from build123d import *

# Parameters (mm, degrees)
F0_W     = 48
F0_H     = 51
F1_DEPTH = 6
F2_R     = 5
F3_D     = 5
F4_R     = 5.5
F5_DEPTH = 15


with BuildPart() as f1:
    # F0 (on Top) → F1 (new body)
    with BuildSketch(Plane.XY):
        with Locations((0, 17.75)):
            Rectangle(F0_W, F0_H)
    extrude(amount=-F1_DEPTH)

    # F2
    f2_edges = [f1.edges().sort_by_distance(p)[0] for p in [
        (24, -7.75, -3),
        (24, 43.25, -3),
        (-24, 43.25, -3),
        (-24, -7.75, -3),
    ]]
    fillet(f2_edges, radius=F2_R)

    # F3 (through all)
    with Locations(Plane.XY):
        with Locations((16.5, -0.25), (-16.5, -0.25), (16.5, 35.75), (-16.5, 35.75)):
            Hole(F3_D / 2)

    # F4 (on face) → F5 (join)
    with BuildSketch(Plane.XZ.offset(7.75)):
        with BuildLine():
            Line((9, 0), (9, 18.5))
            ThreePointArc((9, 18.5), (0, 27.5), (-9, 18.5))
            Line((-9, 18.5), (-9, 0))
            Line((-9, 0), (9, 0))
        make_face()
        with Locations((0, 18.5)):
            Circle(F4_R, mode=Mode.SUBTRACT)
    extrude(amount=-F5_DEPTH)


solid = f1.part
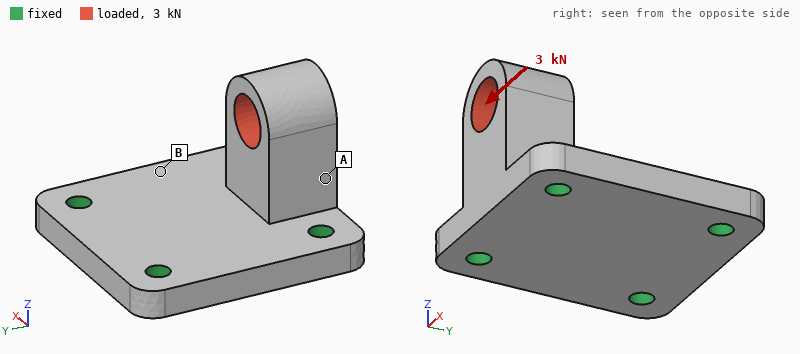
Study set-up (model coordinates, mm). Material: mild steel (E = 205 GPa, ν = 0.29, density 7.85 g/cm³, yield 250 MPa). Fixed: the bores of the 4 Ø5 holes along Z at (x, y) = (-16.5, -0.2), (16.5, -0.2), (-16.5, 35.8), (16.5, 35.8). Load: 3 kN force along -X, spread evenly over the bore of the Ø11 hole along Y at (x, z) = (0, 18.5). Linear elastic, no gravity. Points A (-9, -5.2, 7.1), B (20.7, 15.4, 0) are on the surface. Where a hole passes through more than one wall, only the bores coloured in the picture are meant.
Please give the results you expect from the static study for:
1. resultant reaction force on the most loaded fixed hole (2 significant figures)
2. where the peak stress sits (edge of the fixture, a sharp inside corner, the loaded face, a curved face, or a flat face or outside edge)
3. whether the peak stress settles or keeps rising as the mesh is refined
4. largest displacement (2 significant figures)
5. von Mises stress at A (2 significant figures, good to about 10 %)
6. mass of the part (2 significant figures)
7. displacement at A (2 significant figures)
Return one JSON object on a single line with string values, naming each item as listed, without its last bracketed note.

{"resultant reaction force on the most loaded fixed hole": "2.8 kN", "where the peak stress sits": "edge of the fixture", "whether the peak stress settles or keeps rising as the mesh is refined": "keeps rising", "largest displacement": "33 µm", "von Mises stress at A": "47 MPa", "mass of the part": "150 g", "displacement at A": "9.5 µm"}
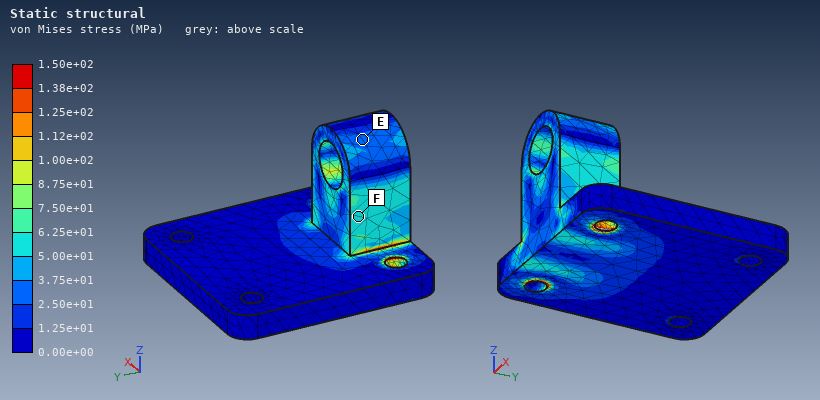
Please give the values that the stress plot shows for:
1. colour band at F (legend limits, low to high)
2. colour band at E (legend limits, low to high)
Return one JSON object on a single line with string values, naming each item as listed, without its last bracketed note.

{"colour band at F": "5.00e+01 to 6.25e+01 MPa", "colour band at E": "2.50e+01 to 3.75e+01 MPa"}
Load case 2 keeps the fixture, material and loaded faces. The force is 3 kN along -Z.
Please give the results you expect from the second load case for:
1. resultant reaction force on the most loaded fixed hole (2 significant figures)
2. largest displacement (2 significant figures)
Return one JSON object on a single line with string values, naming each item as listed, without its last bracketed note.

{"resultant reaction force on the most loaded fixed hole": "1.5 kN", "largest displacement": "8.7 µm"}
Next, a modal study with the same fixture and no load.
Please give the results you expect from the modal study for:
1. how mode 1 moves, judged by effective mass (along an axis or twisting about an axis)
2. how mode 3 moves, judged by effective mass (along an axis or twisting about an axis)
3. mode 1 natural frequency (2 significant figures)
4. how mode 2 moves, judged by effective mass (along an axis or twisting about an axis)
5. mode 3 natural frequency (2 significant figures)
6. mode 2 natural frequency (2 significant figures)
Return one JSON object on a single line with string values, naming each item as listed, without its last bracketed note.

{"how mode 1 moves, judged by effective mass": "along Y", "how mode 3 moves, judged by effective mass": "along Z", "mode 1 natural frequency": "7600 Hz", "how mode 2 moves, judged by effective mass": "along X", "mode 3 natural frequency": "16 kHz", "mode 2 natural frequency": "12 kHz"}
